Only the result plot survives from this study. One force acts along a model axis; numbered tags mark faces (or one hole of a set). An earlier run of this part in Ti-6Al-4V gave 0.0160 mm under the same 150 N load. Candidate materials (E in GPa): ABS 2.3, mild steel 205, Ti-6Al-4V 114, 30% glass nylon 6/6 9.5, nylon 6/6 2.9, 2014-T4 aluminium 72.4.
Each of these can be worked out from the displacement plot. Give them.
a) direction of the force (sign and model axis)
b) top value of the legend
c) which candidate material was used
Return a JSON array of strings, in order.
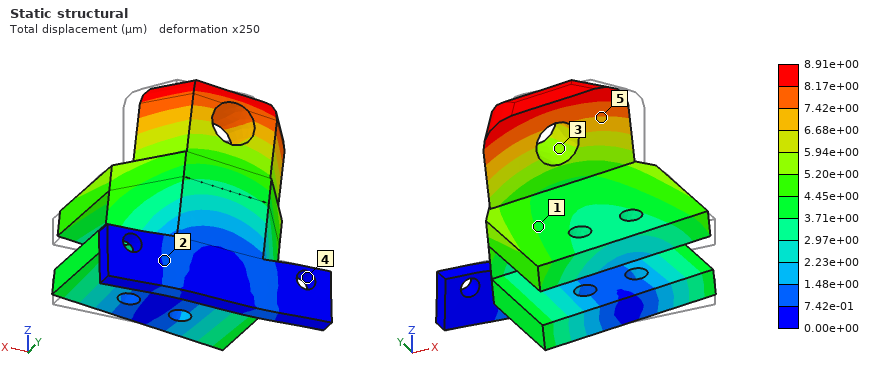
["-X", "8.91e+00 µm", "mild steel"]
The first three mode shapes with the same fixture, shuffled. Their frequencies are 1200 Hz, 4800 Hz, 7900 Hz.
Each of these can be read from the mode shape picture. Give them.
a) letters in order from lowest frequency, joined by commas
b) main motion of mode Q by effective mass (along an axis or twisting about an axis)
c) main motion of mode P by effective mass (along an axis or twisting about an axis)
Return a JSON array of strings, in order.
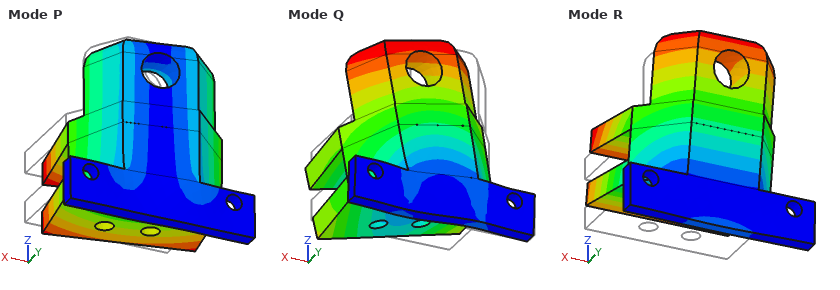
["R, P, Q", "along X", "along X"]
